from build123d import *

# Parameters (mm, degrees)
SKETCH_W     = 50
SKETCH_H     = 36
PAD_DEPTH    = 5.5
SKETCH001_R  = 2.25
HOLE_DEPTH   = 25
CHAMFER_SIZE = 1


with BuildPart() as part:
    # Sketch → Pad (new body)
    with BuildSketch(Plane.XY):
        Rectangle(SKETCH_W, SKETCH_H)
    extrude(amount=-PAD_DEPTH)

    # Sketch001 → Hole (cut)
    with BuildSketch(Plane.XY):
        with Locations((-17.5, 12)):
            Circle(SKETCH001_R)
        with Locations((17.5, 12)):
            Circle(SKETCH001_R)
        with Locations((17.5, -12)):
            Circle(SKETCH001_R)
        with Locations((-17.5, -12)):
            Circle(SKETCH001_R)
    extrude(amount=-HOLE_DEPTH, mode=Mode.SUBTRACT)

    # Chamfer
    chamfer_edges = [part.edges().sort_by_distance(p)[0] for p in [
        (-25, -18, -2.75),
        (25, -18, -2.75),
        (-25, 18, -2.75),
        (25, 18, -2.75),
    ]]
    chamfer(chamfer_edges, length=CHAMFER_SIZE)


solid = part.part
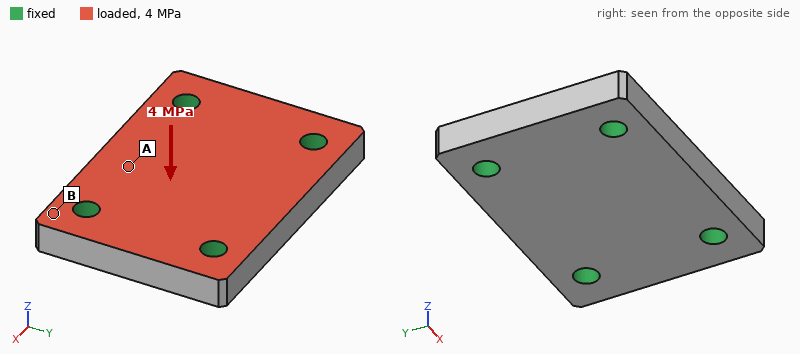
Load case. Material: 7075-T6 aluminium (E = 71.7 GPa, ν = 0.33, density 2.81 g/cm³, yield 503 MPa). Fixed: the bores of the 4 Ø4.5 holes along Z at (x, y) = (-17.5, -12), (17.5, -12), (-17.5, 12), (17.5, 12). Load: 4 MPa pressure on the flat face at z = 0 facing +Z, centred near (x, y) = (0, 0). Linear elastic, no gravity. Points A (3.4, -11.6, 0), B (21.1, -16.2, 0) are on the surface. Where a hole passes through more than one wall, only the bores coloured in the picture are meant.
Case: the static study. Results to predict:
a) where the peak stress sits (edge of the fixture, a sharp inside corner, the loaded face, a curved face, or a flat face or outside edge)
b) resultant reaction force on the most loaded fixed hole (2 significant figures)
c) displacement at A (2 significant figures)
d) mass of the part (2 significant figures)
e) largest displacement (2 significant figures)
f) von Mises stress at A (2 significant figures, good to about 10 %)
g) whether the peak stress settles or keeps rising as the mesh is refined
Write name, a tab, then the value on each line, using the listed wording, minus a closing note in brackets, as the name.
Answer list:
where the peak stress sits	edge of the fixture
resultant reaction force on the most loaded fixed hole	1.7 kN
displacement at A	18 µm
mass of the part	27 g
largest displacement	22 µm
von Mises stress at A	32 MPa
whether the peak stress settles or keeps rising as the mesh is refined	keeps rising
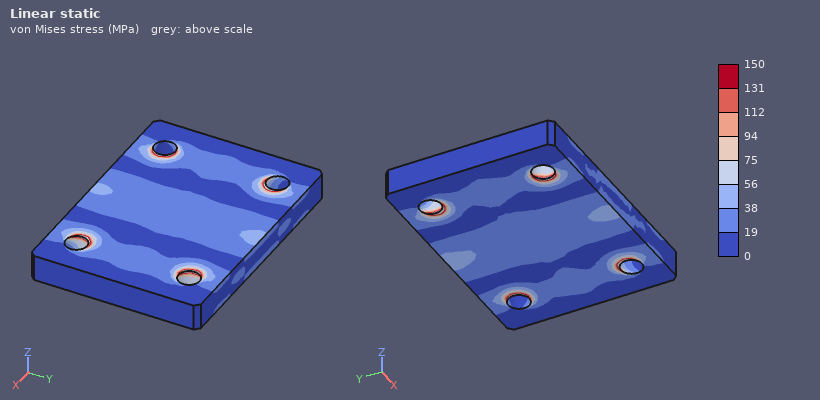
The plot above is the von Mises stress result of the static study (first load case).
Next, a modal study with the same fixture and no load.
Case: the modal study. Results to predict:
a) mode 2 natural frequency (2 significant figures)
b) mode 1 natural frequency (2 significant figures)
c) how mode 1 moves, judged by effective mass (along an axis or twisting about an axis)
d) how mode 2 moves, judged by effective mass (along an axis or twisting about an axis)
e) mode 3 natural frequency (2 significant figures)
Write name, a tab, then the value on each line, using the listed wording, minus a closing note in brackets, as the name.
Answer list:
mode 2 natural frequency	25 kHz
mode 1 natural frequency	20 kHz
how mode 1 moves, judged by effective mass	along Z
how mode 2 moves, judged by effective mass	twisting about X
mode 3 natural frequency	34 kHz
